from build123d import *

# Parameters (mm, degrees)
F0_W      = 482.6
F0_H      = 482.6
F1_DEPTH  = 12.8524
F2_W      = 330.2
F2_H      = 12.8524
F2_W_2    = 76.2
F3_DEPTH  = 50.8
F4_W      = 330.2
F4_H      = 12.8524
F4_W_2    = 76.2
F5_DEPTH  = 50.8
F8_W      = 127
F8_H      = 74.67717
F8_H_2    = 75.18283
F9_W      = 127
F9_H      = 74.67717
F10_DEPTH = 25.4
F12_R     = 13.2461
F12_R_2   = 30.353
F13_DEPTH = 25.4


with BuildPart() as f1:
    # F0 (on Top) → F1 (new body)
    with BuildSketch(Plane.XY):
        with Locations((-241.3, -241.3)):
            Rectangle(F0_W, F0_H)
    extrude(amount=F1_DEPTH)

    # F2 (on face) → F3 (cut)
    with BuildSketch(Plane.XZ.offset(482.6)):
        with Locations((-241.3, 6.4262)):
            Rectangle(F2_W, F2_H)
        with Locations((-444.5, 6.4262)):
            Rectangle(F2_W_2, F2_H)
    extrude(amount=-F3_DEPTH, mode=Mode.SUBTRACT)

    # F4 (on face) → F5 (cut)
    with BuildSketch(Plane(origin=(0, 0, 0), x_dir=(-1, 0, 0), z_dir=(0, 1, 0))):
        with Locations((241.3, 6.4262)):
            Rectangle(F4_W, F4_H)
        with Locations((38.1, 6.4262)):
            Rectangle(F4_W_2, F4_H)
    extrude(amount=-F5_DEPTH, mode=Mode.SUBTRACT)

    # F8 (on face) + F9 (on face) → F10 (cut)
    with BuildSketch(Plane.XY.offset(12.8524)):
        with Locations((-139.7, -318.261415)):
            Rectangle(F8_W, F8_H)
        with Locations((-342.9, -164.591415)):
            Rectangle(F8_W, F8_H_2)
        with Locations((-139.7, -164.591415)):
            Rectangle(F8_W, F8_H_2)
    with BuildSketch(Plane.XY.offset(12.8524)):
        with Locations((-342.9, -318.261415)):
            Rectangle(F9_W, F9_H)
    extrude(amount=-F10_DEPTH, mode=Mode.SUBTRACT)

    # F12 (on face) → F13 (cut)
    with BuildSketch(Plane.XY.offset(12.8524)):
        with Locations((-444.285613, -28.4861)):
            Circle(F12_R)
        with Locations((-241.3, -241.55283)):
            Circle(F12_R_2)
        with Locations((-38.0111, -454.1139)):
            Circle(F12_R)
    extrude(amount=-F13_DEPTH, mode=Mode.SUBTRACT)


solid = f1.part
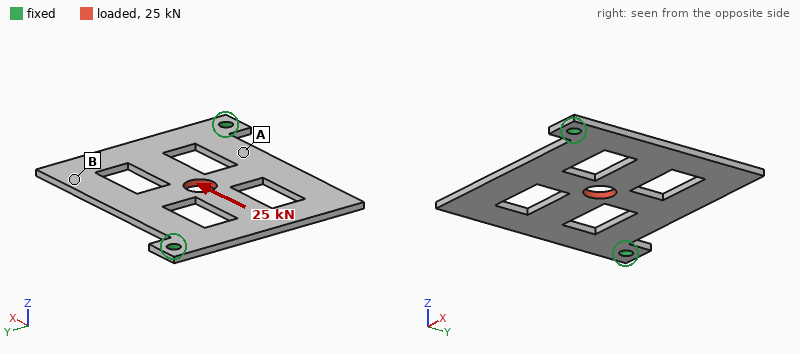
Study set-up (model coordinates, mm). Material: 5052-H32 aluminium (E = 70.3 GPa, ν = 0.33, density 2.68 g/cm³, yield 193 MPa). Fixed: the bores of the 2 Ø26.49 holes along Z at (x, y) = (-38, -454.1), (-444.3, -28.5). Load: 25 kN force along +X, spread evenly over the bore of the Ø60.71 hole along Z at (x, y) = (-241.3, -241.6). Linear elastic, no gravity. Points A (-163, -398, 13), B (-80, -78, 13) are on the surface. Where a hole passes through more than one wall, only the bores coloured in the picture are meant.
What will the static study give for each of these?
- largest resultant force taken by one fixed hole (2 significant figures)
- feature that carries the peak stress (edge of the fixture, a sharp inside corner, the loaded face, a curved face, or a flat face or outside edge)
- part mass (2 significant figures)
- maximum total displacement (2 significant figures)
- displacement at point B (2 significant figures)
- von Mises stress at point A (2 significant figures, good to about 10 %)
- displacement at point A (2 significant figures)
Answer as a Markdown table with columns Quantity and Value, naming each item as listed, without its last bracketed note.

| Quantity | Value |
|---|---|
| largest resultant force taken by one fixed hole | 13 kN |
| feature that carries the peak stress | edge of the fixture |
| part mass | 5.2 kg |
| maximum total displacement | 0.14 mm |
| displacement at point B | 0.081 mm |
| von Mises stress at point A | 14 MPa |
| displacement at point A | 0.066 mm |
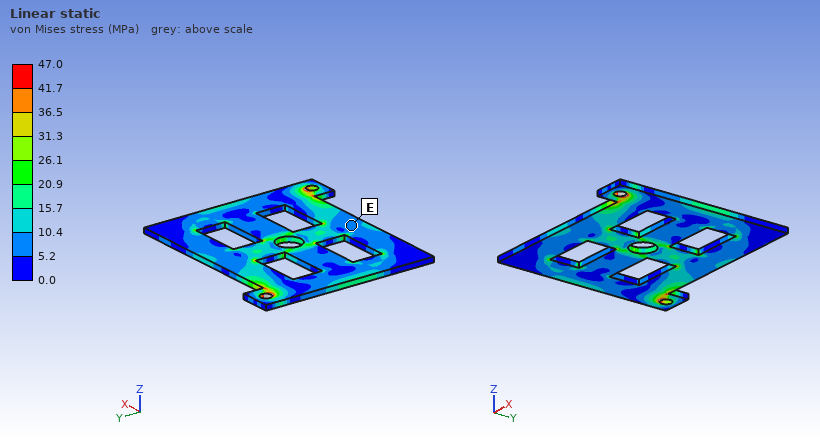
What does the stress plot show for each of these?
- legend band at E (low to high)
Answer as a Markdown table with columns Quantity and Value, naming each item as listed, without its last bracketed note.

| Quantity | Value |
|---|---|
| legend band at E | 5.2 to 10.4 MPa |
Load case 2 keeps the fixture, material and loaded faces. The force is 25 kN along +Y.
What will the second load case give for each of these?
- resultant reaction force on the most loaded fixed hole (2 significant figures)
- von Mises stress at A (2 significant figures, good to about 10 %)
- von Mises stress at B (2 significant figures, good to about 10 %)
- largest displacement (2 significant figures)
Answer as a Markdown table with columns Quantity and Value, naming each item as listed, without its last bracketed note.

| Quantity | Value |
|---|---|
| resultant reaction force on the most loaded fixed hole | 13 kN |
| von Mises stress at A | 12 MPa |
| von Mises stress at B | 4.5 MPa |
| largest displacement | 0.14 mm |
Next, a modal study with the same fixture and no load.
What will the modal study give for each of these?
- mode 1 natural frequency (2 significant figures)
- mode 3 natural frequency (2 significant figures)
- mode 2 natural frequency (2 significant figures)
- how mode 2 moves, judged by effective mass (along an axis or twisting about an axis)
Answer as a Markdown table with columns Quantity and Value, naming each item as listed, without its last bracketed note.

| Quantity | Value |
|---|---|
| mode 1 natural frequency | 85 Hz |
| mode 3 natural frequency | 280 Hz |
| mode 2 natural frequency | 110 Hz |
| how mode 2 moves, judged by effective mass | along Z |
